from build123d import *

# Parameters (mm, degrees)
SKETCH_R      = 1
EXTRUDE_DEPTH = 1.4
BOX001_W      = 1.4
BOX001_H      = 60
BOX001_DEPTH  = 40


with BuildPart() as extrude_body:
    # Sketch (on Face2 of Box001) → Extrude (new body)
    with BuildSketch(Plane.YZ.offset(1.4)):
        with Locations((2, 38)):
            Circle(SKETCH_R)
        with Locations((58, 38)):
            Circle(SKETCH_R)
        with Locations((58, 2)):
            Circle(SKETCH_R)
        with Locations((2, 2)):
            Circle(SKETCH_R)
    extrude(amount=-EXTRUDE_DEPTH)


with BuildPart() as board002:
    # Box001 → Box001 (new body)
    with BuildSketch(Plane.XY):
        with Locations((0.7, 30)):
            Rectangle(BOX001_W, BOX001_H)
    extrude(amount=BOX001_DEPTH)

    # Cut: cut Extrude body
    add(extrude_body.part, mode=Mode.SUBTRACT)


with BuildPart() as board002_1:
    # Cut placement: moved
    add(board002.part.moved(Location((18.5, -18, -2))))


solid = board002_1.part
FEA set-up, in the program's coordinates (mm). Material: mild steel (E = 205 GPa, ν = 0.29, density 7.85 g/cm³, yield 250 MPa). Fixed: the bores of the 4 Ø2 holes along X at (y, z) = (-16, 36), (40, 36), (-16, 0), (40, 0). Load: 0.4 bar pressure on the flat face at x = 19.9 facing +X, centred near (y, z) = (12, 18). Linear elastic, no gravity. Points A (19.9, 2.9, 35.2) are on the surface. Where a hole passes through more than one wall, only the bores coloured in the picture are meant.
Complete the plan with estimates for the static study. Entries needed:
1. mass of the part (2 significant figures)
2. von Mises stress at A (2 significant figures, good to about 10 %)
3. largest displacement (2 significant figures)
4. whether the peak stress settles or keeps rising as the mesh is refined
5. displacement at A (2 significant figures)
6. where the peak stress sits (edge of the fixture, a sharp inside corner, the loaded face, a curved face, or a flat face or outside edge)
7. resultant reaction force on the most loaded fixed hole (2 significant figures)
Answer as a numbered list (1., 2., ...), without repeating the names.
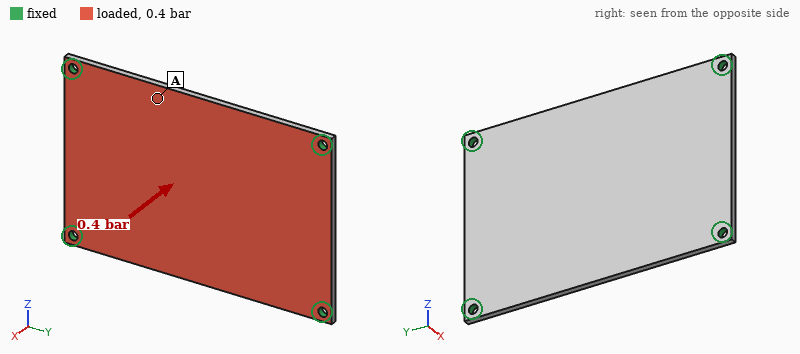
1. 26 g
2. 17 MPa
3. 37 µm
4. keeps rising
5. 28 µm
6. edge of the fixture
7. 24 N
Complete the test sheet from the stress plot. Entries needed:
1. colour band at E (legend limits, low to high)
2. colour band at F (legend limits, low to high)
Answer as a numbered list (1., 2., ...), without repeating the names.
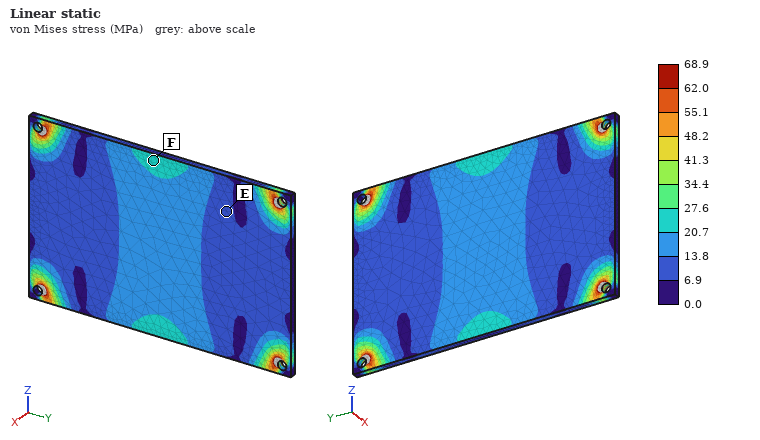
1. 6.9 to 13.8 MPa
2. 20.7 to 27.6 MPa
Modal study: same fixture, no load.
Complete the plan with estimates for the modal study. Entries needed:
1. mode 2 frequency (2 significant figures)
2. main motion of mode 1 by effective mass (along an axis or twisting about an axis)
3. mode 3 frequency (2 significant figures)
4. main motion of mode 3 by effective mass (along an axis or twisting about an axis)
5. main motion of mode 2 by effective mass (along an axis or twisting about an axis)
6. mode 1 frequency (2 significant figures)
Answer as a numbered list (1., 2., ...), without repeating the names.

1. 3200 Hz
2. along X
3. 4600 Hz
4. twisting about Z
5. twisting about Y
6. 1800 Hz
